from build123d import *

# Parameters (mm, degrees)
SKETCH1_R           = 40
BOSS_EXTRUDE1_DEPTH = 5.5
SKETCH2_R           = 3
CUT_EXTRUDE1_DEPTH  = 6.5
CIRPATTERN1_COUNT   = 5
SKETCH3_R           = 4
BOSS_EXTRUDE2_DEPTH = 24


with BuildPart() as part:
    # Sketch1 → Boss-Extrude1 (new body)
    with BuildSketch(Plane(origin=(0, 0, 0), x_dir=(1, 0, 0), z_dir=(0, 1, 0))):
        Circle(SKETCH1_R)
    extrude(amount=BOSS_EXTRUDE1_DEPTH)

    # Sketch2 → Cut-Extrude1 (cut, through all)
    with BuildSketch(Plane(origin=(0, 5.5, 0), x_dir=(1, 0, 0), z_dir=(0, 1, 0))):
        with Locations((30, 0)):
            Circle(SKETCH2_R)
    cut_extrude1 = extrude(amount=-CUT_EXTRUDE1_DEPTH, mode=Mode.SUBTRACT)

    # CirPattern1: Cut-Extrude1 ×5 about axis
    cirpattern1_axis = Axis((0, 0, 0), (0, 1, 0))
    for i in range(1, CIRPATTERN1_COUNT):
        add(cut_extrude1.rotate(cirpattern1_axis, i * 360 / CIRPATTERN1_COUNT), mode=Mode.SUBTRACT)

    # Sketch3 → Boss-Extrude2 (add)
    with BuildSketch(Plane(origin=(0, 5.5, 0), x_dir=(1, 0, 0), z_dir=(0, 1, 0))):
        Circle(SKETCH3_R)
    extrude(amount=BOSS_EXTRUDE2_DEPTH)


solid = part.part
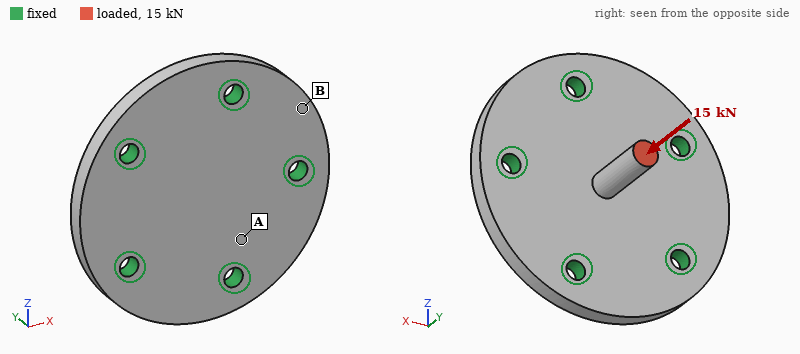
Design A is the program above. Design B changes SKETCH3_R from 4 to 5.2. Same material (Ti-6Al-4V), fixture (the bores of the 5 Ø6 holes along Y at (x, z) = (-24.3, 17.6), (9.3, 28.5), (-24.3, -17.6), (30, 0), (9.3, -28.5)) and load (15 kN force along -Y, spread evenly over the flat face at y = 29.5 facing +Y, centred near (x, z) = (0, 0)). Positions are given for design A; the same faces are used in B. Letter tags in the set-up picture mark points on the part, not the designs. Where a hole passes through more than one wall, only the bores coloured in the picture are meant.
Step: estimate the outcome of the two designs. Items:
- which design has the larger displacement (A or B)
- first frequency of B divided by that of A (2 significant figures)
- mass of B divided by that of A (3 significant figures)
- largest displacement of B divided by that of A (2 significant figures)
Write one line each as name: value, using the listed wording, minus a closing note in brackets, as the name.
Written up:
which design has the larger displacement: A
first frequency of B divided by that of A: 1.1
mass of B divided by that of A: 1.03
largest displacement of B divided by that of A: 0.82
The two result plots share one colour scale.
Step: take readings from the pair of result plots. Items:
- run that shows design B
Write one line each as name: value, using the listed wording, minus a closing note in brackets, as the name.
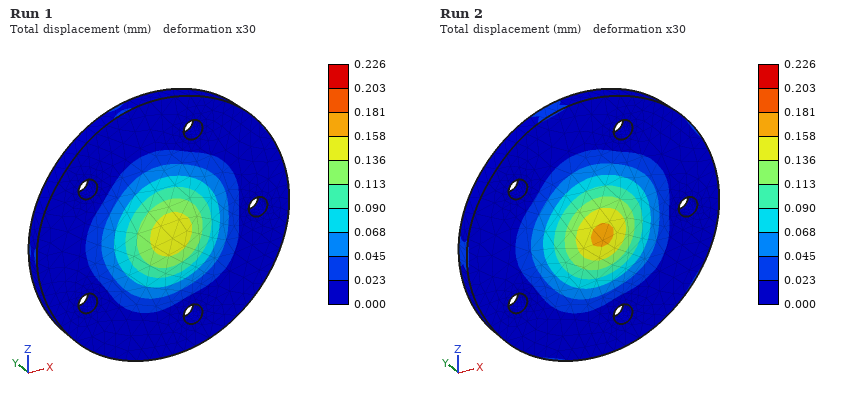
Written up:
run that shows design B: Run 1
